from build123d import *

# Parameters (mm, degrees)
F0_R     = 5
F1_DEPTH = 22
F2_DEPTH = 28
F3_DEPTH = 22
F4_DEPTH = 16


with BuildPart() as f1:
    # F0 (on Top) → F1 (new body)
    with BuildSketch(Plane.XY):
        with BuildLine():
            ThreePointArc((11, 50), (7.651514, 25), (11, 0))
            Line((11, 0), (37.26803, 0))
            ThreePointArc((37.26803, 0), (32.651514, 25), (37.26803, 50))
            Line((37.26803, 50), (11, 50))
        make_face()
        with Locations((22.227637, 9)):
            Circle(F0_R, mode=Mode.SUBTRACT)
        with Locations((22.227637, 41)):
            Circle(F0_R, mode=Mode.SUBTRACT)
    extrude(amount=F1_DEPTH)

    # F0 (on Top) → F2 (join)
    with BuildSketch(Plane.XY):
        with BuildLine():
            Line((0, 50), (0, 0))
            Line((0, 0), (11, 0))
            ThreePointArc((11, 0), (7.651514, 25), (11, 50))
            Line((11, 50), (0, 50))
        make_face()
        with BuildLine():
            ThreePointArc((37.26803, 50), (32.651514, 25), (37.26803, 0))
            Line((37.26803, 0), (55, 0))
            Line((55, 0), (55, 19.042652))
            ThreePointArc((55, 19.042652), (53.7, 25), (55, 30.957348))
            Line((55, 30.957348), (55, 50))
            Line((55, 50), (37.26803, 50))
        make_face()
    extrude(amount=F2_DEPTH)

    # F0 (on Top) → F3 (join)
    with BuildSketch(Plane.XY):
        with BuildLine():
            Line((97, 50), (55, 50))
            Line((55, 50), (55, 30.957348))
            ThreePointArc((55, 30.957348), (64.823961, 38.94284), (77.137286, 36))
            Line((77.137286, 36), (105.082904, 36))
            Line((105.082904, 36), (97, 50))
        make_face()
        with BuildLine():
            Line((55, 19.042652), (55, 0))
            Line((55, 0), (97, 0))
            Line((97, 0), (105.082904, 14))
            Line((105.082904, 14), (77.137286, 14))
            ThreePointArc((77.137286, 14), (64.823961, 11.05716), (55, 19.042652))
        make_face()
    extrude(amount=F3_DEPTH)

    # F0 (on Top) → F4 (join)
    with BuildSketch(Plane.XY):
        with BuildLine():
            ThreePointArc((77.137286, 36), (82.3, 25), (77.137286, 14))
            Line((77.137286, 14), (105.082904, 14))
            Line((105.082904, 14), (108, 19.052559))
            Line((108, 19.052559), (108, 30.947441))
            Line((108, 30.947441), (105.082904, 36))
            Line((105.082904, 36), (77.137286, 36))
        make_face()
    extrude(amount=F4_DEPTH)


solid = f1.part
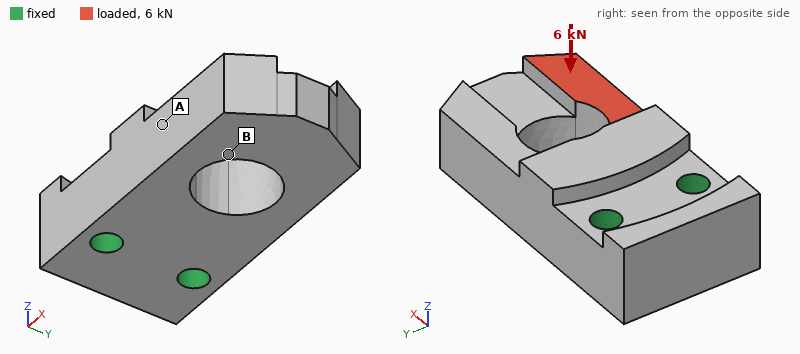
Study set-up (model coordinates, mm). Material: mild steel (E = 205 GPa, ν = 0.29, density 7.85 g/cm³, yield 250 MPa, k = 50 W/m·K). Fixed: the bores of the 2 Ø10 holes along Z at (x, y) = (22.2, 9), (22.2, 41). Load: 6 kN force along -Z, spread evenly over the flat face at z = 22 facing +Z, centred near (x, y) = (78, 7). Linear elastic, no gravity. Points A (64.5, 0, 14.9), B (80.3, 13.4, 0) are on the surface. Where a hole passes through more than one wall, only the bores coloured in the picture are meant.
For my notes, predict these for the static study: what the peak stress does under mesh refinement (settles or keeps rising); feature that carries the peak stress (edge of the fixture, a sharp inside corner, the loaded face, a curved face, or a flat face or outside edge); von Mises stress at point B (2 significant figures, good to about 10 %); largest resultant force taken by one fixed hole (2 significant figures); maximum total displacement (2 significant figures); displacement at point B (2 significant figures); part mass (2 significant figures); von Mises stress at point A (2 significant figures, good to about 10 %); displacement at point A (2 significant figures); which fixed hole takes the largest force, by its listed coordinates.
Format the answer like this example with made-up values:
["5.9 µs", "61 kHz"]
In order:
["keeps rising", "edge of the fixture", "22 MPa", "5.4 kN", "90 µm", "55 µm", "800 g", "55 MPa", "35 µm", "(22.2, 9)"]
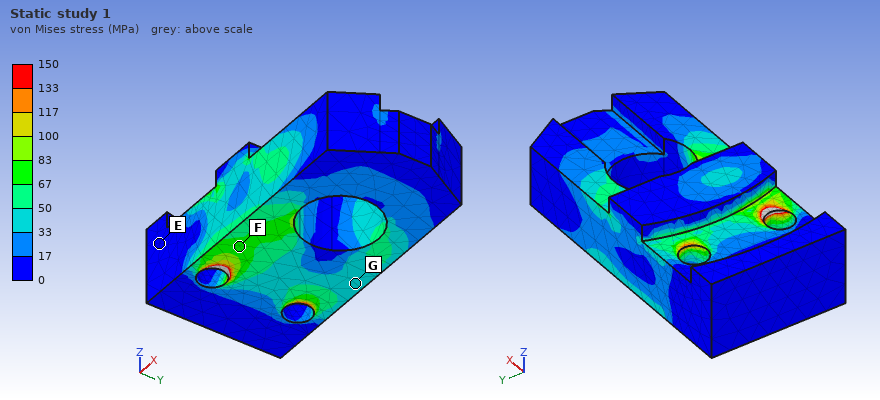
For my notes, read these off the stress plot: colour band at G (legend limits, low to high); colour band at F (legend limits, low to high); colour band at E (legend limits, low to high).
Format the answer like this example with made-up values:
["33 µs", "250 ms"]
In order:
["33 to 50 MPa", "67 to 83 MPa", "0 to 17 MPa"]
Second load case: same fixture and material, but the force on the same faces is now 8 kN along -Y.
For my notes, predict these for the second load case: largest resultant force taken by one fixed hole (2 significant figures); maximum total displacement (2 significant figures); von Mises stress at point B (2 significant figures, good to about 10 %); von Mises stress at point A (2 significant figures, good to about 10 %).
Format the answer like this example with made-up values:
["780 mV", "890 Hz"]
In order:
["13 kN", "53 µm", "27 MPa", "63 MPa"]
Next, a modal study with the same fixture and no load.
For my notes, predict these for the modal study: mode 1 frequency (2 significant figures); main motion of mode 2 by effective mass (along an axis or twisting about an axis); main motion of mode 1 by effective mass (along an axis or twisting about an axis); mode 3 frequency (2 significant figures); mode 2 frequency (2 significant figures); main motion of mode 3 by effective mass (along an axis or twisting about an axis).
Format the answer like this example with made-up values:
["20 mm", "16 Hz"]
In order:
["2800 Hz", "along Y", "along Z", "6900 Hz", "4600 Hz", "twisting about X"]
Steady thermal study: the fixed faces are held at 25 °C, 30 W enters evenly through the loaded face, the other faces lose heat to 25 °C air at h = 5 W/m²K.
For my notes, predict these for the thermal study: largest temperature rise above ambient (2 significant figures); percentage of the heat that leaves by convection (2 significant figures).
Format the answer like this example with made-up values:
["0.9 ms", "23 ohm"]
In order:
["55 K", "5.0 %"]
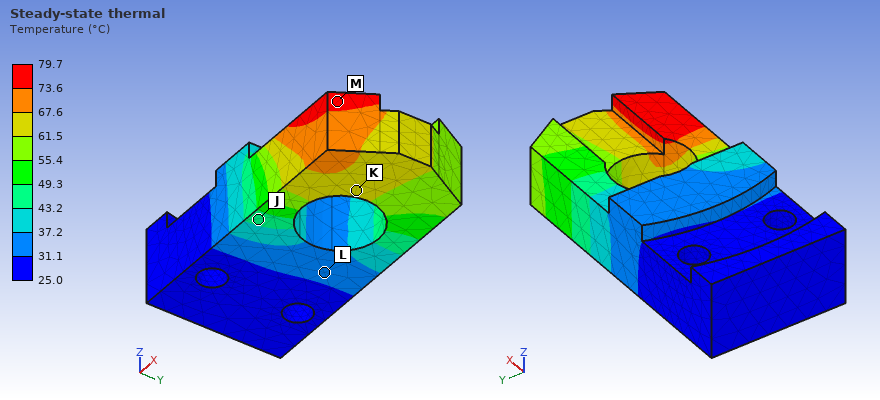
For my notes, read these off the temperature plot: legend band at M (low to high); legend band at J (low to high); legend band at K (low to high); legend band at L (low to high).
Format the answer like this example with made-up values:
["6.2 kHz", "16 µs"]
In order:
["73.6 to 79.7 °C", "43.2 to 49.3 °C", "61.5 to 67.6 °C", "31.1 to 37.2 °C"]
